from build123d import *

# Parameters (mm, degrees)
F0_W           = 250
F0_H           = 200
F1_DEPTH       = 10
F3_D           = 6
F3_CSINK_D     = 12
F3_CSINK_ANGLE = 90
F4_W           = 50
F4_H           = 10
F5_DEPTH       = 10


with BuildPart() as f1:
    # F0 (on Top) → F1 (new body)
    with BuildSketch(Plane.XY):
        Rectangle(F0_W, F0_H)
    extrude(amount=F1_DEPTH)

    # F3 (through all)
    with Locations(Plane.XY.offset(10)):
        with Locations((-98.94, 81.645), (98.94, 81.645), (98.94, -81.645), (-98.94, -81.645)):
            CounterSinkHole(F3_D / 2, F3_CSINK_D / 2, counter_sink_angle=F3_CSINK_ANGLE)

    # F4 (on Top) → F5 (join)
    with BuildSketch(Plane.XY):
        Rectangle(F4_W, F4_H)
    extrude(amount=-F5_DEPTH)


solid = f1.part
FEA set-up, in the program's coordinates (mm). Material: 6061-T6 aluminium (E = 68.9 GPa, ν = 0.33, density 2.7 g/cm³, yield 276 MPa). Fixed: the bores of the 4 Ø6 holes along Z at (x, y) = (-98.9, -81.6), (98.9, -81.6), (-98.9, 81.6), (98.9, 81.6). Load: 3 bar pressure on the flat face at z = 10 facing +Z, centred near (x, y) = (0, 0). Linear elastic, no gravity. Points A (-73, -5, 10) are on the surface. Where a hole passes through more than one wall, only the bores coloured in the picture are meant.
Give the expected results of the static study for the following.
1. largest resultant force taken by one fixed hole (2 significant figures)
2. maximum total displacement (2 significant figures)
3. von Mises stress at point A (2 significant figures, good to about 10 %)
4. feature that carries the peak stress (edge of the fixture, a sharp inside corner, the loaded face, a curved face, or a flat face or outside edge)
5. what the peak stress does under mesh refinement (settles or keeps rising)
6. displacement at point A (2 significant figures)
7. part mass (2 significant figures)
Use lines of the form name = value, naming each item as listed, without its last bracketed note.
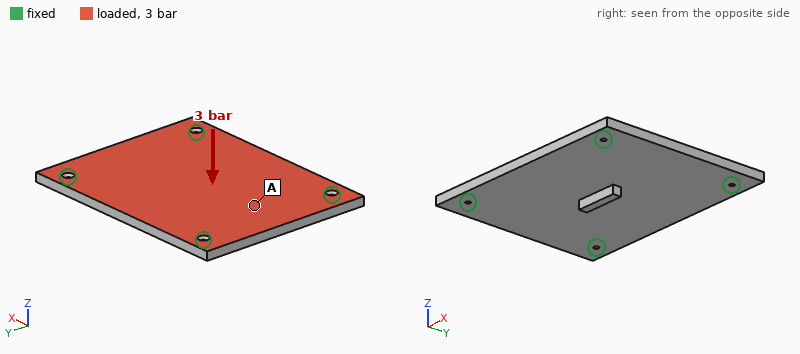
largest resultant force taken by one fixed hole = 4.2 kN
maximum total displacement = 0.50 mm
von Mises stress at point A = 32 MPa
feature that carries the peak stress = edge of the fixture
what the peak stress does under mesh refinement = keeps rising
displacement at point A = 0.33 mm
part mass = 1.4 kg
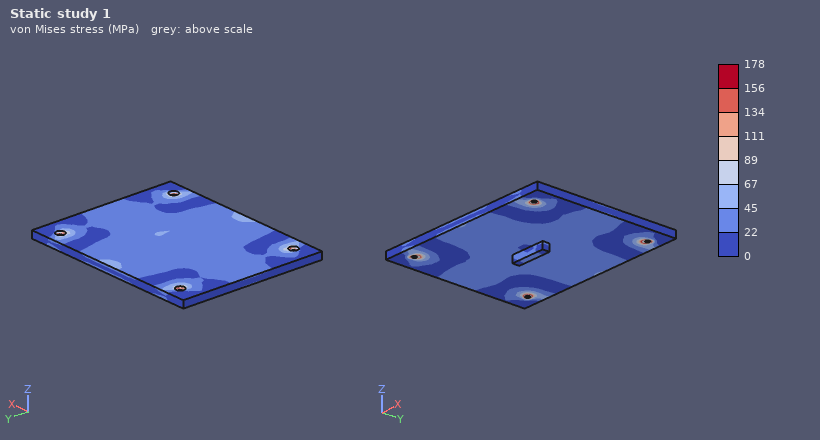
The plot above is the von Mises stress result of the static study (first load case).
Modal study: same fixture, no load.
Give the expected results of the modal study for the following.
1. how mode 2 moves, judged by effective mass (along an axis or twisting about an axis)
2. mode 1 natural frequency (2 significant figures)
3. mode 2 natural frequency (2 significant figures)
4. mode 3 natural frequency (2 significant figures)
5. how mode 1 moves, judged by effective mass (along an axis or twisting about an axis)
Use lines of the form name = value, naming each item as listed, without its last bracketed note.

how mode 2 moves, judged by effective mass = twisting about X
mode 1 natural frequency = 860 Hz
mode 2 natural frequency = 1400 Hz
mode 3 natural frequency = 1600 Hz
how mode 1 moves, judged by effective mass = along Z
